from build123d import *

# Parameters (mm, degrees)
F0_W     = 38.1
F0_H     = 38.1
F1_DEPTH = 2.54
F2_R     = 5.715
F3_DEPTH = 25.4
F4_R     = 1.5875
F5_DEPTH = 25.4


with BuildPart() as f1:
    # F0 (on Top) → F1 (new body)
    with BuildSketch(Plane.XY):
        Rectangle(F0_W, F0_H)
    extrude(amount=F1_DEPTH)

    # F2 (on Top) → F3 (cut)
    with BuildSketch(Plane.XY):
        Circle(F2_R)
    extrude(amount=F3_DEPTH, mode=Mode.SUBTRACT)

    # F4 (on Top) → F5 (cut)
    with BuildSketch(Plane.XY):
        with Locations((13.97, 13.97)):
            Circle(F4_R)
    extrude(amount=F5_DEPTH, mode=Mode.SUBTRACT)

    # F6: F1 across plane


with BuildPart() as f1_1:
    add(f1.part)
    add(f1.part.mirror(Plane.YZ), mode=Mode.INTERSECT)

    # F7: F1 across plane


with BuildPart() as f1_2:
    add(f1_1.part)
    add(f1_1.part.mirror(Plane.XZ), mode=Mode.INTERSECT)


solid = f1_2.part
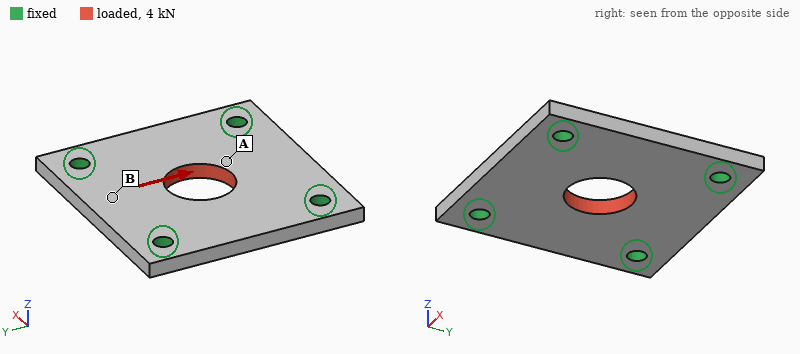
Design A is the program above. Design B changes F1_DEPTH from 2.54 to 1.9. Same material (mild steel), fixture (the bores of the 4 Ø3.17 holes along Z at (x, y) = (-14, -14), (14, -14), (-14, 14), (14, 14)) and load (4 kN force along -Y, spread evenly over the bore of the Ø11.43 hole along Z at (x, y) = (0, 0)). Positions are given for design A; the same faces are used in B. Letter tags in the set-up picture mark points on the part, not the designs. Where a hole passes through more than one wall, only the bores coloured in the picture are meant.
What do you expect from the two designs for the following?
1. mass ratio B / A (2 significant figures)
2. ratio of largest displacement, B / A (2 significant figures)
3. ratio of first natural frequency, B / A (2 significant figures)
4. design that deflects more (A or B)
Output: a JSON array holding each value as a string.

["0.75", "1.3", "0.78", "B"]
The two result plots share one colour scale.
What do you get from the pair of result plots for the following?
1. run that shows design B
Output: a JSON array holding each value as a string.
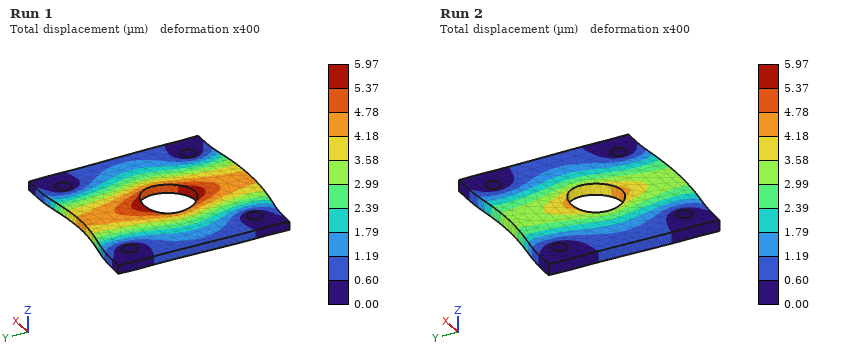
["Run 1"]
